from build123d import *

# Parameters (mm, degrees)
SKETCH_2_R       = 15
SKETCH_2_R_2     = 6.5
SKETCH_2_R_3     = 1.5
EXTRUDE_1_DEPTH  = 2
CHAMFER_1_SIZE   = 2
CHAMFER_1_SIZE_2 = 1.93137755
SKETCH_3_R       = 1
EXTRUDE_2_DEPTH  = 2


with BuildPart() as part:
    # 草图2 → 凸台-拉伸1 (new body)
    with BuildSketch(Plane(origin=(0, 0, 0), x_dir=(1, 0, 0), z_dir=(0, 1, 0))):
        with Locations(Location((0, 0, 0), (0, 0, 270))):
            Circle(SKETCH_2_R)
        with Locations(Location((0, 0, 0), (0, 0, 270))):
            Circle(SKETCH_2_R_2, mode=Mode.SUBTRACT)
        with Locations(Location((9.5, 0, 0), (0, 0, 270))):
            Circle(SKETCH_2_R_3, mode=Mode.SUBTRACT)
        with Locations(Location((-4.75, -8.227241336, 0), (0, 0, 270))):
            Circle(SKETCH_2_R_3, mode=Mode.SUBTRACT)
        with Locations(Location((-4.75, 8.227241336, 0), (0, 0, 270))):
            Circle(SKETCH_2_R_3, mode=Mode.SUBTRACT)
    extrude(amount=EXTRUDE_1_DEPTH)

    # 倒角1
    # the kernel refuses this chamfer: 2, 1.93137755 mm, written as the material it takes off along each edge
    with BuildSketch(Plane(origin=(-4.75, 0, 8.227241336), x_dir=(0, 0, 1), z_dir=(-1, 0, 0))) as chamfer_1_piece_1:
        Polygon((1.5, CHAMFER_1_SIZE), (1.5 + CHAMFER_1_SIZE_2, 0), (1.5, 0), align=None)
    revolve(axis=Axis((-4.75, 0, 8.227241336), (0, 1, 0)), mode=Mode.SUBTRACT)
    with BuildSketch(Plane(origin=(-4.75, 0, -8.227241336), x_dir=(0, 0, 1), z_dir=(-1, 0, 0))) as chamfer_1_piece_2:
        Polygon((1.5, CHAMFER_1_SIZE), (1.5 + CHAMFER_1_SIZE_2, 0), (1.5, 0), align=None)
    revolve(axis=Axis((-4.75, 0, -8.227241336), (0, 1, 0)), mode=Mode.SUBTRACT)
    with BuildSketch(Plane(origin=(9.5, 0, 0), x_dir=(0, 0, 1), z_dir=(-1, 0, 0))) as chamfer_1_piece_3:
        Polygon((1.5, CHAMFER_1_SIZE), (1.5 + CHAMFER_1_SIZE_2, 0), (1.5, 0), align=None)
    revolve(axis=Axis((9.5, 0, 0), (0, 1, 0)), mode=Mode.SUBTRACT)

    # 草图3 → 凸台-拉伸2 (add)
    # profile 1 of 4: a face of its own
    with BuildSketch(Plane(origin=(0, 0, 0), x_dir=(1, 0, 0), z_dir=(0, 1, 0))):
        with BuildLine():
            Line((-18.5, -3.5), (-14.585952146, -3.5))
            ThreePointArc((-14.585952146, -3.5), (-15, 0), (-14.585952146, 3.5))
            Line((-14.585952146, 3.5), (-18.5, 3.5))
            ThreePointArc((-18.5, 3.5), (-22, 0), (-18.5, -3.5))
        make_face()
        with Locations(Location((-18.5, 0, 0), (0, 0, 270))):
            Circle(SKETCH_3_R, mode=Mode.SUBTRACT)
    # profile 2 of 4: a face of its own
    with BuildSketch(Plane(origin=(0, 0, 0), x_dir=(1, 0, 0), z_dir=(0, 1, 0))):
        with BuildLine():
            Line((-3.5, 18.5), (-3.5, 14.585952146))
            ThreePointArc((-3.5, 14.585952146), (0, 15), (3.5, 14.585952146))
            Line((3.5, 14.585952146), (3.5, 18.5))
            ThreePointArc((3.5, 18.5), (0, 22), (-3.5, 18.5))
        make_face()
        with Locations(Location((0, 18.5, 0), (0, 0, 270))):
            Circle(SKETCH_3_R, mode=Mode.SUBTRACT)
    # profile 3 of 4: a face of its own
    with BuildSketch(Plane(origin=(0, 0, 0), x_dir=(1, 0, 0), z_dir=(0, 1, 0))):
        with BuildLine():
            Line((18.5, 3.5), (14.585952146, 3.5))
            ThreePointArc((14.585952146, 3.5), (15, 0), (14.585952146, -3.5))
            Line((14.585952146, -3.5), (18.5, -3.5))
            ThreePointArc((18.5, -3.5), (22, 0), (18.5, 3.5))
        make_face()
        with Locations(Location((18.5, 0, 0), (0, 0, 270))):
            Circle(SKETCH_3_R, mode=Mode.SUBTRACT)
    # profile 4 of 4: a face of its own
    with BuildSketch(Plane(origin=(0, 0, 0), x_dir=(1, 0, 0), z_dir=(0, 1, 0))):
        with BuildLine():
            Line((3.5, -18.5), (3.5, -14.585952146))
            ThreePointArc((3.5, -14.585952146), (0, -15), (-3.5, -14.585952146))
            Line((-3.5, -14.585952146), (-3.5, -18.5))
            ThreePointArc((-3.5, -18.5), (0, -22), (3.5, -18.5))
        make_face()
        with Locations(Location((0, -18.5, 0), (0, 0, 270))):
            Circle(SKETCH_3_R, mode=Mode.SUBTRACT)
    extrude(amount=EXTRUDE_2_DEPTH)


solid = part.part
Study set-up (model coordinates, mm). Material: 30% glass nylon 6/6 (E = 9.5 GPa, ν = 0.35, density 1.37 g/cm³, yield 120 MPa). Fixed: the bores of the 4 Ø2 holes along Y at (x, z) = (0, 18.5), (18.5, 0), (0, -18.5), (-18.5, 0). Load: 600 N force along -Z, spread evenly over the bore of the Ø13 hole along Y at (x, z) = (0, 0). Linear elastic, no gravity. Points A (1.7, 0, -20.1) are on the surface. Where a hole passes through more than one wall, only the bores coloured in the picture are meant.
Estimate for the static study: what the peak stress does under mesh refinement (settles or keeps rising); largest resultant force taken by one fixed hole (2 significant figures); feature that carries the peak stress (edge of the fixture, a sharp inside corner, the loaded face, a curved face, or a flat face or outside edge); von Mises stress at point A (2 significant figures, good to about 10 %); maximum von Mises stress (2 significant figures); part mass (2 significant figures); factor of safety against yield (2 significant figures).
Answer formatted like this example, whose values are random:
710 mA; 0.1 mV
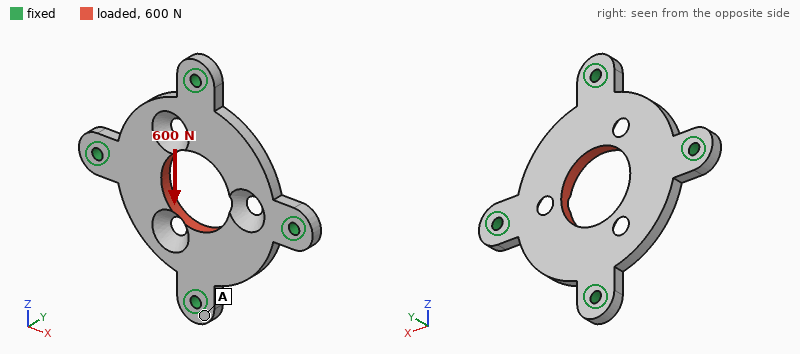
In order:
settles; 220 N; a curved face; 7.0 MPa; 100 MPa; 1.9 g; 1.2
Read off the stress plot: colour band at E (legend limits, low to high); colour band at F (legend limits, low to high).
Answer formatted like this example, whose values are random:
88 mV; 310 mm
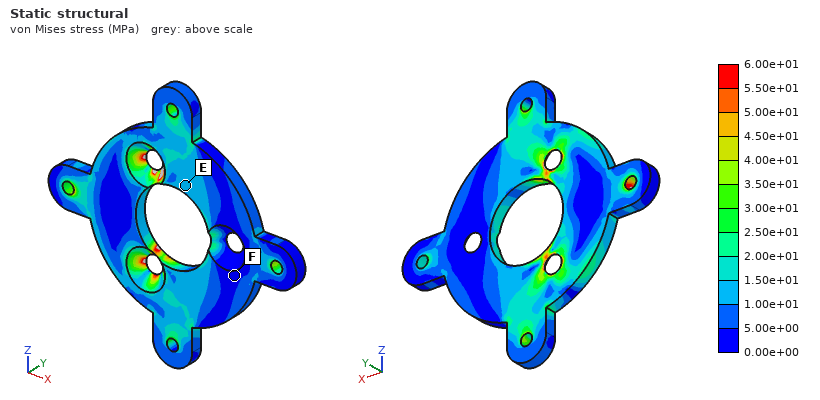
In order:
1.00e+01 to 1.50e+01 MPa; 0.00e+00 to 5.00e+00 MPa
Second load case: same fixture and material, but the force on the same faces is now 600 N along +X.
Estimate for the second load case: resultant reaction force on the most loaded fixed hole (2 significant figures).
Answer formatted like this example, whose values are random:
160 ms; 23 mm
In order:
240 N
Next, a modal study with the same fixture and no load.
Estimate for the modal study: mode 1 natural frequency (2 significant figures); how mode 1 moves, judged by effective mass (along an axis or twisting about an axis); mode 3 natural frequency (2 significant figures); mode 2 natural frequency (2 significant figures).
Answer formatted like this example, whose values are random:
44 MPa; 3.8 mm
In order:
5700 Hz; along Y; 8100 Hz; 7900 Hz
